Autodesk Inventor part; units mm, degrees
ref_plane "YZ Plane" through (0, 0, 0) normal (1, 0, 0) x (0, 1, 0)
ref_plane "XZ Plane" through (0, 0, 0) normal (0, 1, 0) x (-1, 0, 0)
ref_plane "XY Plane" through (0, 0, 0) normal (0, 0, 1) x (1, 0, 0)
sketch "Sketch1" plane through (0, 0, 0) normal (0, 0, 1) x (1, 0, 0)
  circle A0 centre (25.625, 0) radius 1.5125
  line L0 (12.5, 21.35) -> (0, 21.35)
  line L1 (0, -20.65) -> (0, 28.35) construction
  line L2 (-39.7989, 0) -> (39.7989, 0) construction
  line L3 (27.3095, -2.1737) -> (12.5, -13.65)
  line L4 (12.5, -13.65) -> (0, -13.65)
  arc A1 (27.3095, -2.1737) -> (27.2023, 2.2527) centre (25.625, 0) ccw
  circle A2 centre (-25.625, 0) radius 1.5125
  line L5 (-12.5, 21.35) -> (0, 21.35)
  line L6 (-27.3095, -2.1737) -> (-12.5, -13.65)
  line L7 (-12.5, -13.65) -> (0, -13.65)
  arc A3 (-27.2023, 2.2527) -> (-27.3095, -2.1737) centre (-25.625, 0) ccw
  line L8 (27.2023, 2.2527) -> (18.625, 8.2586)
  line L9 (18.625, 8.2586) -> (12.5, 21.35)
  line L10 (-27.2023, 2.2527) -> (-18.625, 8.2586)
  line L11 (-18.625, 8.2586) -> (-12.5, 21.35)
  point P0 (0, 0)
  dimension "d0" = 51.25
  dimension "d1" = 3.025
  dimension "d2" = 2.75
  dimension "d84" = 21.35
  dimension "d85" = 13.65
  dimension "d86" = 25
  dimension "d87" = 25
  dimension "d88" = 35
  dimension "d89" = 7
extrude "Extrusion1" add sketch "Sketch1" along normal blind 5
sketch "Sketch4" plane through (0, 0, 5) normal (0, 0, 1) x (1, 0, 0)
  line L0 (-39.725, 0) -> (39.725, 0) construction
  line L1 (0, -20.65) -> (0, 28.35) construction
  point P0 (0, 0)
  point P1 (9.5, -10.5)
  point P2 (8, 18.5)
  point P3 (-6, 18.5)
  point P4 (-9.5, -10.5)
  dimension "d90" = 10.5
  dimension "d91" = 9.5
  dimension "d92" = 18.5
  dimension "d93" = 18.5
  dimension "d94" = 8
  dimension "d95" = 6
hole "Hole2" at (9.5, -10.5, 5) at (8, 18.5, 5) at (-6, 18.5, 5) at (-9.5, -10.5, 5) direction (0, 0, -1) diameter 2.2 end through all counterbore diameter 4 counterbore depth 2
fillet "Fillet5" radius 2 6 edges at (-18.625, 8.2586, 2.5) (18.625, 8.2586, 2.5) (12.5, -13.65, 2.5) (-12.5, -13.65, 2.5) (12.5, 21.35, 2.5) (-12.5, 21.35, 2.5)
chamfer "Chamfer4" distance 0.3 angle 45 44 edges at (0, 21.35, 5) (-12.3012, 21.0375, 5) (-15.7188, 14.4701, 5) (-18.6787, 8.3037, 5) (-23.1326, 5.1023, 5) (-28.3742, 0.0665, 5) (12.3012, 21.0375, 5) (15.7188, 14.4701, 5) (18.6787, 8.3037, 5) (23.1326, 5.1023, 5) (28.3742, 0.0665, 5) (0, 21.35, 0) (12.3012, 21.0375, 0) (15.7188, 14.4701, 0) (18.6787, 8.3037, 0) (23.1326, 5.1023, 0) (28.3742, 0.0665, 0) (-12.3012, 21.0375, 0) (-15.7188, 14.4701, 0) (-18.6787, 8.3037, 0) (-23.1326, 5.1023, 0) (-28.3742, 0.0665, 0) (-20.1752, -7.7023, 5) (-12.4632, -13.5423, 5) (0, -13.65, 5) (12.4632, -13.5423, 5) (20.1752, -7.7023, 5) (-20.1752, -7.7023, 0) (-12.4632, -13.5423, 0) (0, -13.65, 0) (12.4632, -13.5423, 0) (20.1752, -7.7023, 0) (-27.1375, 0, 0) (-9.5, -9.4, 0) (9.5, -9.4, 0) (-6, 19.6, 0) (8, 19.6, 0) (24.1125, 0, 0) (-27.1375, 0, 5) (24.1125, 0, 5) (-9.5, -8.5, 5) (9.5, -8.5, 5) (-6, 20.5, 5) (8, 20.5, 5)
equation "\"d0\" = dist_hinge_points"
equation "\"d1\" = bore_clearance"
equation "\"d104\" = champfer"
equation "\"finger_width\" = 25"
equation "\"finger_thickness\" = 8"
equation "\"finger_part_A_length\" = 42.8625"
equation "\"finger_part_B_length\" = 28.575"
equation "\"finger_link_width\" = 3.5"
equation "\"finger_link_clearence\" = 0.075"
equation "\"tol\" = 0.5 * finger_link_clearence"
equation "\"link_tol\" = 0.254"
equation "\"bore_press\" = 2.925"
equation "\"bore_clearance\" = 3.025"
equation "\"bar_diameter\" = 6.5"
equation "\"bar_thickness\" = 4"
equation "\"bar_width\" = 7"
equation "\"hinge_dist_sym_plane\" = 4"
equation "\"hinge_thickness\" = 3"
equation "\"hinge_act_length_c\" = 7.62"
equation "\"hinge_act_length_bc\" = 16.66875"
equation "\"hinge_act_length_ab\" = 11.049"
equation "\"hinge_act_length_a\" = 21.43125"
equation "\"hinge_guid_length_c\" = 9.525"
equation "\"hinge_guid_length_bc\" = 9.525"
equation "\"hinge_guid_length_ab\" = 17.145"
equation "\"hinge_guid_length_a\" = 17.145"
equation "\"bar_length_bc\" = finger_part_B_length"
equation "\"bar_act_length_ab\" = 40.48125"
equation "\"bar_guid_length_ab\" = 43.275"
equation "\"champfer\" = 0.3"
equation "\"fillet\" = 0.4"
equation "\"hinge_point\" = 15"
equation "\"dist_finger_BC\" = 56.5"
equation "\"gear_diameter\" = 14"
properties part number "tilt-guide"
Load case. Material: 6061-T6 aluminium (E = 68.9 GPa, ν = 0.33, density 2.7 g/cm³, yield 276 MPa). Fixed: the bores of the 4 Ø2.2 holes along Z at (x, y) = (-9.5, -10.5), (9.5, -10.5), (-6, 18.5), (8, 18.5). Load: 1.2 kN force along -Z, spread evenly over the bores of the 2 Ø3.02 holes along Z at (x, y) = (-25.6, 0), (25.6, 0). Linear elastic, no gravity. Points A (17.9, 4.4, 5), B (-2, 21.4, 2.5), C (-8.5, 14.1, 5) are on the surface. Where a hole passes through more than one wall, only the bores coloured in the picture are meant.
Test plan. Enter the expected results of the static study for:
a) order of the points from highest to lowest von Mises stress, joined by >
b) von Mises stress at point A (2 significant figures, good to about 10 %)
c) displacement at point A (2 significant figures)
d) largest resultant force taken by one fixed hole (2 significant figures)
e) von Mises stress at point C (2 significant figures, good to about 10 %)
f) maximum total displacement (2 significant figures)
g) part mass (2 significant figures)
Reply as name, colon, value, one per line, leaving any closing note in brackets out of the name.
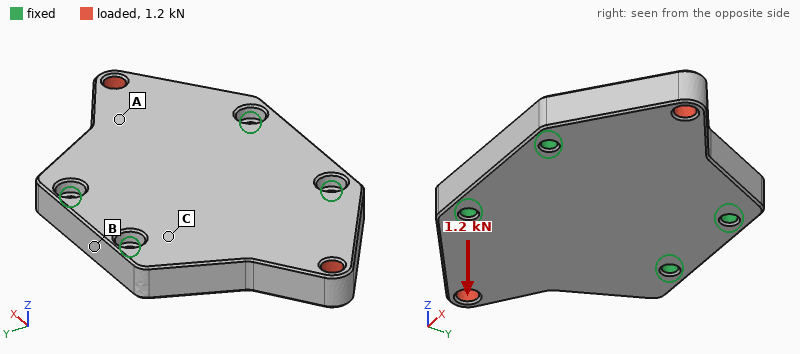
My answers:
order of the points from highest to lowest von Mises stress, joined by >: A > C > B
von Mises stress at point A: 91 MPa
displacement at point A: 0.059 mm
largest resultant force taken by one fixed hole: 680 N
von Mises stress at point C: 55 MPa
maximum total displacement: 0.16 mm
part mass: 18 g
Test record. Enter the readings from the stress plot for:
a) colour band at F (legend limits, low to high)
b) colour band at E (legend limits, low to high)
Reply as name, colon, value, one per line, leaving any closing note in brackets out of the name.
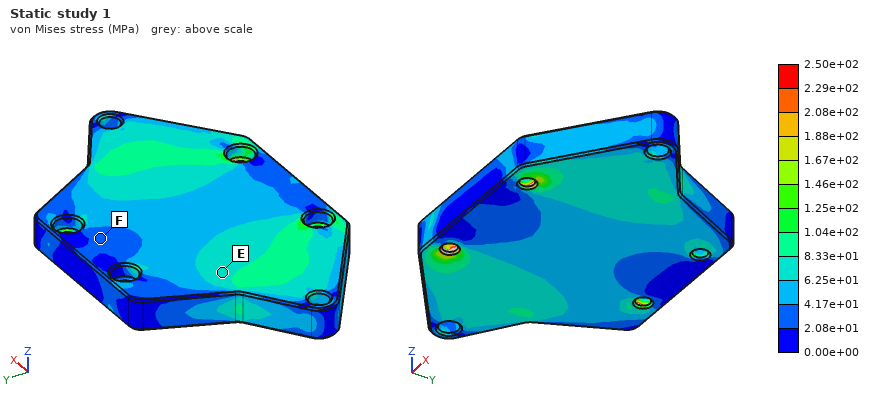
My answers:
colour band at F: 2.08e+01 to 4.17e+01 MPa
colour band at E: 6.25e+01 to 8.33e+01 MPa
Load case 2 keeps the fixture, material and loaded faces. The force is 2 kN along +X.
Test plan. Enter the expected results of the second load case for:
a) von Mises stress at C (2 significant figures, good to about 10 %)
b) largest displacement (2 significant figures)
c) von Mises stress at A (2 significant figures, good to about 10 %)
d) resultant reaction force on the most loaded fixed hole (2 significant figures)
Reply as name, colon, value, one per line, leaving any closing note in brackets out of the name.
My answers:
von Mises stress at C: 8.4 MPa
largest displacement: 9.4 µm
von Mises stress at A: 13 MPa
resultant reaction force on the most loaded fixed hole: 630 N
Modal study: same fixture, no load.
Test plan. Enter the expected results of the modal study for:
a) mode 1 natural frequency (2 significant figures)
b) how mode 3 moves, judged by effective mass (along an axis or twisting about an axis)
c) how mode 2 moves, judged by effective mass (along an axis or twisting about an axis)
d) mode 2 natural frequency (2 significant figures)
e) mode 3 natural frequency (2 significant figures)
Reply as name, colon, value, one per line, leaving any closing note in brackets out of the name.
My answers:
mode 1 natural frequency: 10 kHz
how mode 3 moves, judged by effective mass: along Z
how mode 2 moves, judged by effective mass: along Z
mode 2 natural frequency: 11 kHz
mode 3 natural frequency: 21 kHz
